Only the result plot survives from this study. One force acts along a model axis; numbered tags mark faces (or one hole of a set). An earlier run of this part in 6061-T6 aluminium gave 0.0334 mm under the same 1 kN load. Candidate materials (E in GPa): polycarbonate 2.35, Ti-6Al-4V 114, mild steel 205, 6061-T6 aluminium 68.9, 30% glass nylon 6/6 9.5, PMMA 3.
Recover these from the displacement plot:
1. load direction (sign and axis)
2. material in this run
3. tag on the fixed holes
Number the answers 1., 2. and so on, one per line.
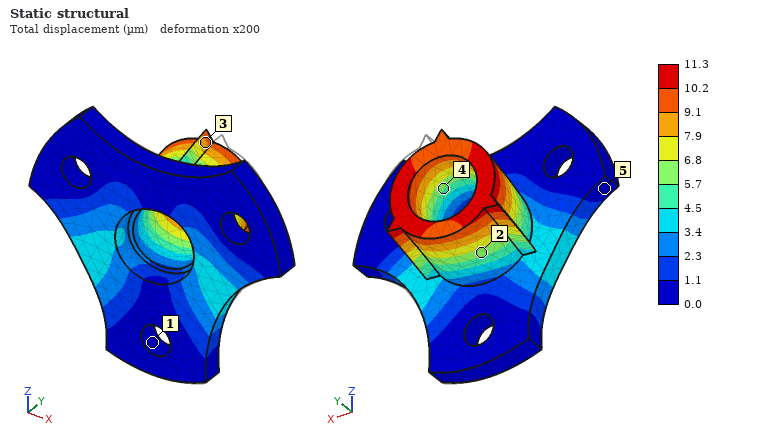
1. -X
2. mild steel
3. 1
